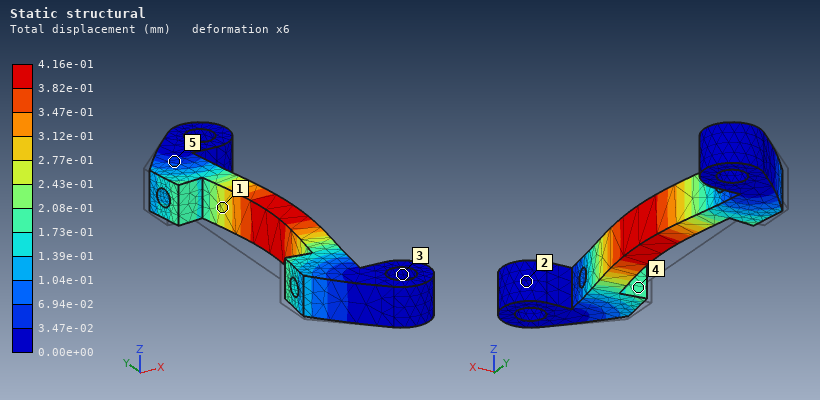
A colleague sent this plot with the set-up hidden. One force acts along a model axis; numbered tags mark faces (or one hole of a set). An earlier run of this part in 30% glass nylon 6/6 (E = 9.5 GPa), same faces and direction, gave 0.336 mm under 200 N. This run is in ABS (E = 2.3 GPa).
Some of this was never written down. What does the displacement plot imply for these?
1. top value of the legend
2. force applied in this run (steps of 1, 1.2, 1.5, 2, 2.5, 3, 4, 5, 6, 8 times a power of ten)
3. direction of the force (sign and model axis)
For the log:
4.16e-01 mm
60 N
+X
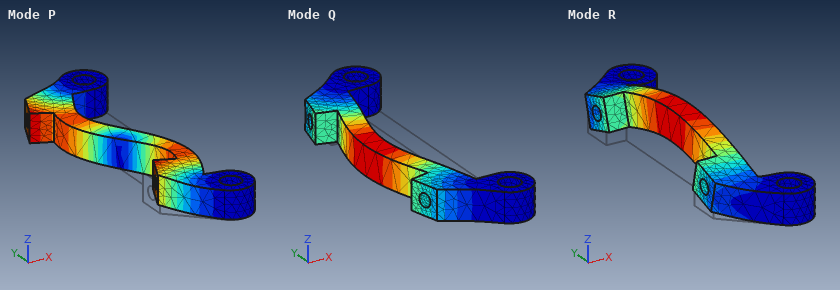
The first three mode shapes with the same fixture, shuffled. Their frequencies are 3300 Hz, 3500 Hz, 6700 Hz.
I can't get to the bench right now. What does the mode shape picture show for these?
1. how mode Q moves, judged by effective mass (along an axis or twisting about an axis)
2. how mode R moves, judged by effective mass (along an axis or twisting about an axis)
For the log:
along X
along Z
